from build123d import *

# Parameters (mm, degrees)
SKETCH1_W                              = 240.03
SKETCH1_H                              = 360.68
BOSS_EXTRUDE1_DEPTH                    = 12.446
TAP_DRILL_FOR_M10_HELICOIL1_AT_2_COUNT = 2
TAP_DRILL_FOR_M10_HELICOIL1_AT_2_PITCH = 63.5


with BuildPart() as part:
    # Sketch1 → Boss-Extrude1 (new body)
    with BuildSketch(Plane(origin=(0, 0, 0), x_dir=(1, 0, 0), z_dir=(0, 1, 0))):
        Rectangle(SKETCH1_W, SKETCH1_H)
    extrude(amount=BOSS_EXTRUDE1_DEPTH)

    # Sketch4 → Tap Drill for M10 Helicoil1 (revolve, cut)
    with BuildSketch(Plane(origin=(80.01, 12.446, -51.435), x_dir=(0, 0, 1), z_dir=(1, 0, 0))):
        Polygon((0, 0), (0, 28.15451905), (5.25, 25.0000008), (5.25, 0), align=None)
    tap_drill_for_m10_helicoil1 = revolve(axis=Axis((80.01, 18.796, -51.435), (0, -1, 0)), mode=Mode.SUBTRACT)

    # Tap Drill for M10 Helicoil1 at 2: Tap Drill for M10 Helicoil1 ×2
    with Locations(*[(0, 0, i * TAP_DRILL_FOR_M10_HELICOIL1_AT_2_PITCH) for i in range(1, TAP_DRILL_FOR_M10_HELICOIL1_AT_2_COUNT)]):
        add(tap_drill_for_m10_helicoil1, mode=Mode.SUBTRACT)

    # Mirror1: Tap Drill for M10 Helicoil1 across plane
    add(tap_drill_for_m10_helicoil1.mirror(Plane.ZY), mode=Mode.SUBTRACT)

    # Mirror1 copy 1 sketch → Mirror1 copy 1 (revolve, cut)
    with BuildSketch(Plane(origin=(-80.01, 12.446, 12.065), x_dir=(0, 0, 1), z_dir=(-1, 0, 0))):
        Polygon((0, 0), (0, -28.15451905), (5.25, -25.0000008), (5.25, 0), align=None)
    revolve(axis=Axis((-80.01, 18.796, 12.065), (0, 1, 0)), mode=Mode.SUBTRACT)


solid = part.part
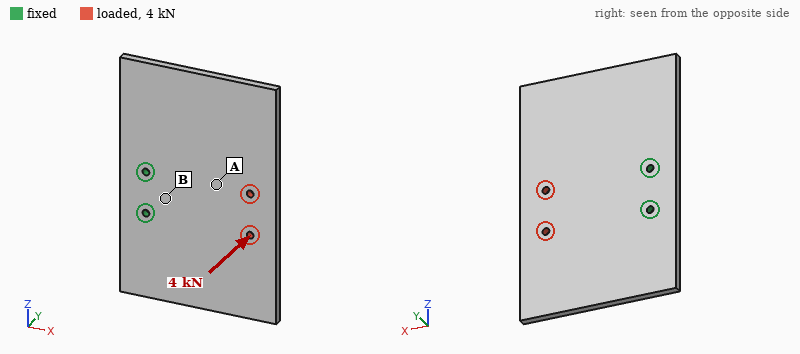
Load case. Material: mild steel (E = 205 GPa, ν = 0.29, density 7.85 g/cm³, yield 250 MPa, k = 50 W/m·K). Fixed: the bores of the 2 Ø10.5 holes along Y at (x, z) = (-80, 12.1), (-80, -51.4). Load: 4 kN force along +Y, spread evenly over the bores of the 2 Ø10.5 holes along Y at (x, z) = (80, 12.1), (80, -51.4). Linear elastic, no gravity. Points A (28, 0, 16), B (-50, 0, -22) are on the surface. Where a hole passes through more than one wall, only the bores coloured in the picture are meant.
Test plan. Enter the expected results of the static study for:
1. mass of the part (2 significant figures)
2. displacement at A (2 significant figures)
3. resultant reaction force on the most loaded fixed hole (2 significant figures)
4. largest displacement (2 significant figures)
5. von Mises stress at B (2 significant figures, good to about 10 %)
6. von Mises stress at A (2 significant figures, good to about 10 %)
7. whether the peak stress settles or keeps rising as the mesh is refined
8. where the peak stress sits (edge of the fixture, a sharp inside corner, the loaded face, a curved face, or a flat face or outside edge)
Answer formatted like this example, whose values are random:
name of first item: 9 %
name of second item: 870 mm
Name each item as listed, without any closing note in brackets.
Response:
mass of the part: 8.4 kg
displacement at A: 0.46 mm
resultant reaction force on the most loaded fixed hole: 2.0 kN
largest displacement: 1.1 mm
von Mises stress at B: 92 MPa
von Mises stress at A: 26 MPa
whether the peak stress settles or keeps rising as the mesh is refined: keeps rising
where the peak stress sits: edge of the fixture
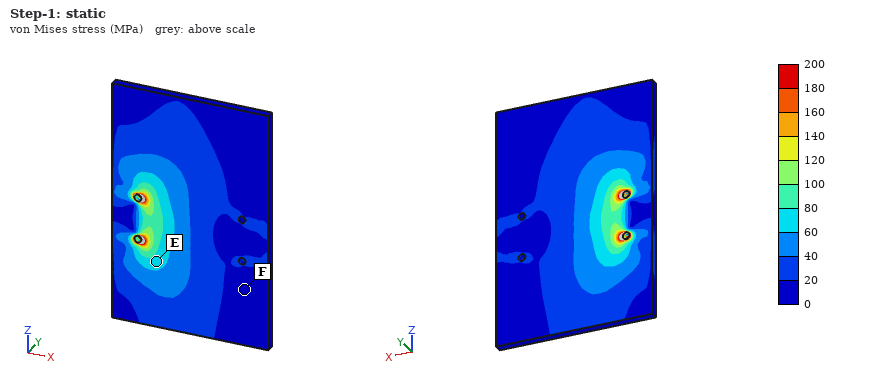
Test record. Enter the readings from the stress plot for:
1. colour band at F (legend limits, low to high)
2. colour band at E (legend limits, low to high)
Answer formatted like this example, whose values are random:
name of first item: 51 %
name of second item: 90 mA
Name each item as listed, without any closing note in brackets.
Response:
colour band at F: 0 to 20 MPa
colour band at E: 60 to 80 MPa
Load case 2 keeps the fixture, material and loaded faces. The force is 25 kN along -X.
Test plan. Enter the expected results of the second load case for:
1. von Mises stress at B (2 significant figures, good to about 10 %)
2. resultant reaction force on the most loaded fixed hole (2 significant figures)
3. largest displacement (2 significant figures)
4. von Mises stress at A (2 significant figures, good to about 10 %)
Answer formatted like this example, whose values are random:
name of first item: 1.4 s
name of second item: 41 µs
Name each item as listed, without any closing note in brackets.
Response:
von Mises stress at B: 12 MPa
resultant reaction force on the most loaded fixed hole: 13 kN
largest displacement: 14 µm
von Mises stress at A: 14 MPa
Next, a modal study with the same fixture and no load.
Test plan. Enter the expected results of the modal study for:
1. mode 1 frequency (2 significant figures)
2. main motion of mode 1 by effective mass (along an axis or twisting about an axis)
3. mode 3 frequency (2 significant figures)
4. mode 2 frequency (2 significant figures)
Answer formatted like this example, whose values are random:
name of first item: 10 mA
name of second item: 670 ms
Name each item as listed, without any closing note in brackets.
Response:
mode 1 frequency: 190 Hz
main motion of mode 1 by effective mass: along Y
mode 3 frequency: 450 Hz
mode 2 frequency: 240 Hz
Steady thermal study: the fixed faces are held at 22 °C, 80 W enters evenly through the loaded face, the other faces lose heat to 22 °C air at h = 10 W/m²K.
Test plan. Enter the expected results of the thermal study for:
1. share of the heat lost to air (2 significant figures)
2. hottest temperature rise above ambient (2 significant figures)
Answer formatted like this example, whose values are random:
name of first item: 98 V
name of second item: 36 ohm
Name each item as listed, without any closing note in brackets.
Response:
share of the heat lost to air: 59 %
hottest temperature rise above ambient: 73 K
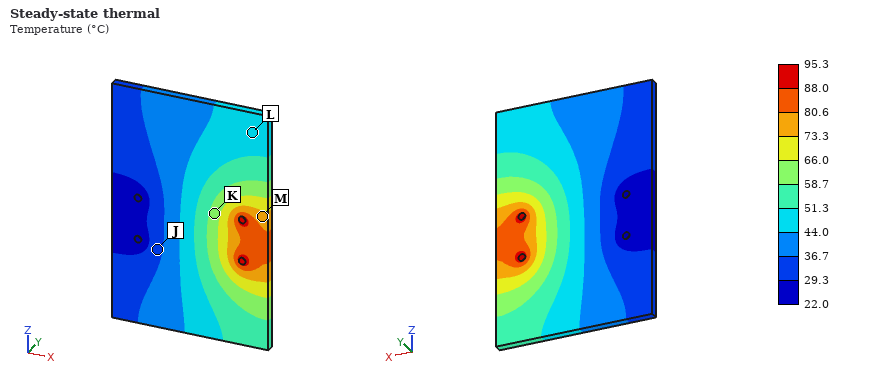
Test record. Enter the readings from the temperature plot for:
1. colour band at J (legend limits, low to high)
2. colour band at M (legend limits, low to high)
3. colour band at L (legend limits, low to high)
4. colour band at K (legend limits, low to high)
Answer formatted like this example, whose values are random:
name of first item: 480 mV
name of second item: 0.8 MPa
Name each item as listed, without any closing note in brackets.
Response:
colour band at J: 29.3 to 36.7 °C
colour band at M: 73.3 to 80.6 °C
colour band at L: 44.0 to 51.3 °C
colour band at K: 58.7 to 66.0 °C
